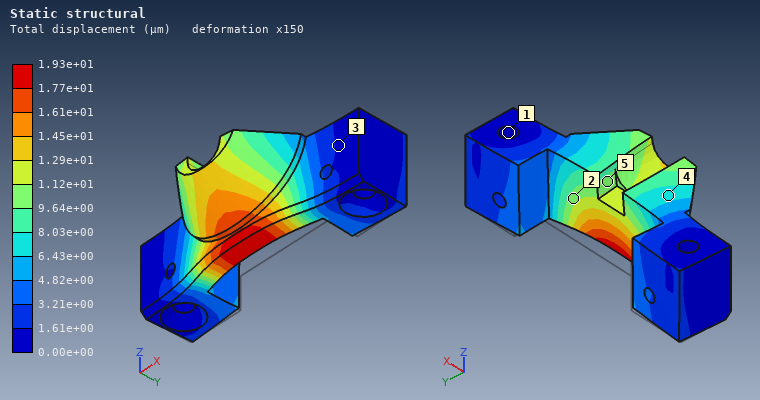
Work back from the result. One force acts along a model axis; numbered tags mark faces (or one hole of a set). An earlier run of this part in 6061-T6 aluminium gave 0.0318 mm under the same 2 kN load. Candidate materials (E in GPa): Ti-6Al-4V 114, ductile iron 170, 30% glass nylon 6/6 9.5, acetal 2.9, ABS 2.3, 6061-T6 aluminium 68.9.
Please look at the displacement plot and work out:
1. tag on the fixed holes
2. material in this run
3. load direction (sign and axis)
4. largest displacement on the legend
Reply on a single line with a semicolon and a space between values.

1; Ti-6Al-4V; -Y; 1.93e+01 µm
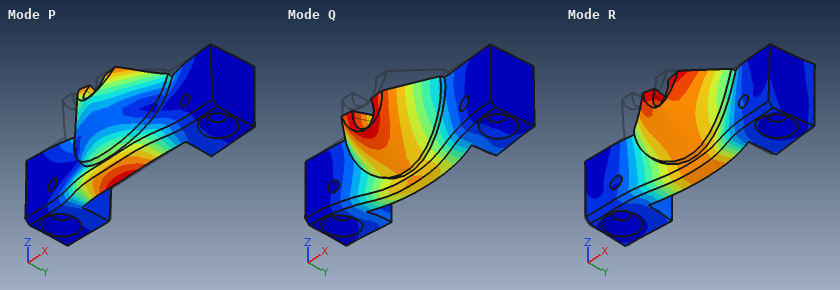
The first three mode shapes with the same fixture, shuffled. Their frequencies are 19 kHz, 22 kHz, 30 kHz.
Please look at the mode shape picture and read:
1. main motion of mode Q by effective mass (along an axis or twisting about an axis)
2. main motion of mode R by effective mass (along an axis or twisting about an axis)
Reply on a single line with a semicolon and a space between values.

along Z; along Y
